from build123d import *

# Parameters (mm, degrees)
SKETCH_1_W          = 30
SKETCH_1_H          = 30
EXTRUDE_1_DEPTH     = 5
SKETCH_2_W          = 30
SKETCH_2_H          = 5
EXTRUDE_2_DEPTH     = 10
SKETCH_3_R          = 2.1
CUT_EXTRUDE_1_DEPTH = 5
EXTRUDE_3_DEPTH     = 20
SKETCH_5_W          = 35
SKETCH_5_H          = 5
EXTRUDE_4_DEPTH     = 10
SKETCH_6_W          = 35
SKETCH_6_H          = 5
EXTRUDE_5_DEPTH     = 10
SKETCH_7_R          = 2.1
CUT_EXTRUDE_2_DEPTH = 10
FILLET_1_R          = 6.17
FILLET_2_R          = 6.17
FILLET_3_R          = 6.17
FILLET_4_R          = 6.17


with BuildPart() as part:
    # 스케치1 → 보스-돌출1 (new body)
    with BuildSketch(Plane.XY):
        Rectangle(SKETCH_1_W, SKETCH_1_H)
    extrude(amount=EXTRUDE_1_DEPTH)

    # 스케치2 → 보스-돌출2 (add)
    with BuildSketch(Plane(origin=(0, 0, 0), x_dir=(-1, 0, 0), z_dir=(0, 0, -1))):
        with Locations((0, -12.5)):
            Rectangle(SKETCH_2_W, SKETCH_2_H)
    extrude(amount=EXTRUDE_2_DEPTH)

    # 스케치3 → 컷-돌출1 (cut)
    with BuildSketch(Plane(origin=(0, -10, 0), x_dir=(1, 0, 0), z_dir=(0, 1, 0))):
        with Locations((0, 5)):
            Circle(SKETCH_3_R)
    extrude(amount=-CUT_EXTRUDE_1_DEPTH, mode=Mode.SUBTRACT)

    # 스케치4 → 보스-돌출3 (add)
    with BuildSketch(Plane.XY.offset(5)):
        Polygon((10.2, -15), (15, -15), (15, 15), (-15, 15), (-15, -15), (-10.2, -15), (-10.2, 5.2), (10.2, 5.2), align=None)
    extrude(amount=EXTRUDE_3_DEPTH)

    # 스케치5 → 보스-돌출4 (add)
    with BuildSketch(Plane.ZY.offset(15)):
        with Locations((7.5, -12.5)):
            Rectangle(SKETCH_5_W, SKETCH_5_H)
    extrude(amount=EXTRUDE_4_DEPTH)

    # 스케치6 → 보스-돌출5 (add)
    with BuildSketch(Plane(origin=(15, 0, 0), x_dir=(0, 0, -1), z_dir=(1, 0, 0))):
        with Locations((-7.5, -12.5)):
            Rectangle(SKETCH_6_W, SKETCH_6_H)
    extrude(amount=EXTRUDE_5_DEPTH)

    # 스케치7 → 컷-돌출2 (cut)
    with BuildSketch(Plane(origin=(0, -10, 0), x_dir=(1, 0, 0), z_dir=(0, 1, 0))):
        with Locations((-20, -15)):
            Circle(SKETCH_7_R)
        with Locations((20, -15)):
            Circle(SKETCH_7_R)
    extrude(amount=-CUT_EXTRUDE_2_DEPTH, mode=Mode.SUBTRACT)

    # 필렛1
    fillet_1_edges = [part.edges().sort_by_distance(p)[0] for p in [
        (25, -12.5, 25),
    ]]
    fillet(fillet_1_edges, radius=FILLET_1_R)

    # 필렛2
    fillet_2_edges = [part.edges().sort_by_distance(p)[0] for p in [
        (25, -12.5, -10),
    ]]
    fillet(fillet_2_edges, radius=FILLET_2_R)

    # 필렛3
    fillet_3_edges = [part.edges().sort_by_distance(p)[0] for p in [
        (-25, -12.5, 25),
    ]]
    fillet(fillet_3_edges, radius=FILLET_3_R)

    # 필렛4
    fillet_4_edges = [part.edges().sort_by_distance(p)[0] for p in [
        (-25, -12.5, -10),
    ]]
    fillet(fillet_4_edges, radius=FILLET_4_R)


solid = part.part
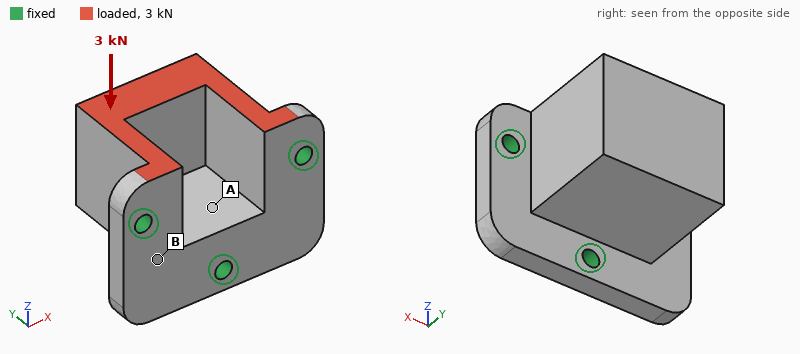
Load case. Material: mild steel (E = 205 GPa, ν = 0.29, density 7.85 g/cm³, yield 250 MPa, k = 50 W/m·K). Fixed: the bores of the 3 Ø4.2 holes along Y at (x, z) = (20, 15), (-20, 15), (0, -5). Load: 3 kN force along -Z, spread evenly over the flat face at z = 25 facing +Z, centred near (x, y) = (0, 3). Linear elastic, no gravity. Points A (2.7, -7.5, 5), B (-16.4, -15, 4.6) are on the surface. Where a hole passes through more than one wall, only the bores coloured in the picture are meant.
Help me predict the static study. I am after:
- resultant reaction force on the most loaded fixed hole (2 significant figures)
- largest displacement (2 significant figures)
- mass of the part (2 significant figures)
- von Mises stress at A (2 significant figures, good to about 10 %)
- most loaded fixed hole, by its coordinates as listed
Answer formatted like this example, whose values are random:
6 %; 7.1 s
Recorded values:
2.3 kN; 20 µm; 150 g; 28 MPa; (0, -5)
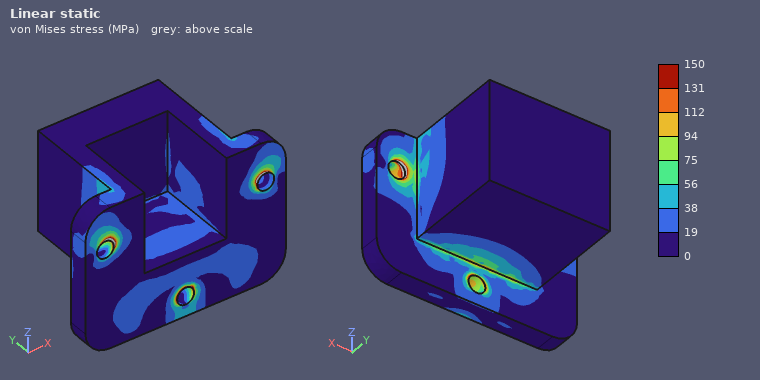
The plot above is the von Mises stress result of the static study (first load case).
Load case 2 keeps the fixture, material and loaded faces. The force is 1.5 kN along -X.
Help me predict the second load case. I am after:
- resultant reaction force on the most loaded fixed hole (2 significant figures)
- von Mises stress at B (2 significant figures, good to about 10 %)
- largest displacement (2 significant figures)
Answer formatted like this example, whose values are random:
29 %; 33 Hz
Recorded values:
910 N; 9.8 MPa; 15 µm
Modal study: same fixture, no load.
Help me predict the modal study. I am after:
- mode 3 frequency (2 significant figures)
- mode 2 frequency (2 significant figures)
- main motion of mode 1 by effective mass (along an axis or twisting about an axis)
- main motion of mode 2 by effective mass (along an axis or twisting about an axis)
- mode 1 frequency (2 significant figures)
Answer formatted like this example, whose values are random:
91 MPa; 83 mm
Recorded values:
13 kHz; 7400 Hz; along Z; along X; 6700 Hz
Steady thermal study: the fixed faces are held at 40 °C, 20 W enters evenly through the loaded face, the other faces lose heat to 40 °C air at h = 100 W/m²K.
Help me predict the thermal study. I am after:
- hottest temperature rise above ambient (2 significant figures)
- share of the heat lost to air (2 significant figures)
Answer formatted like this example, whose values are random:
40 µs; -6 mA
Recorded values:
25 K; 34 %
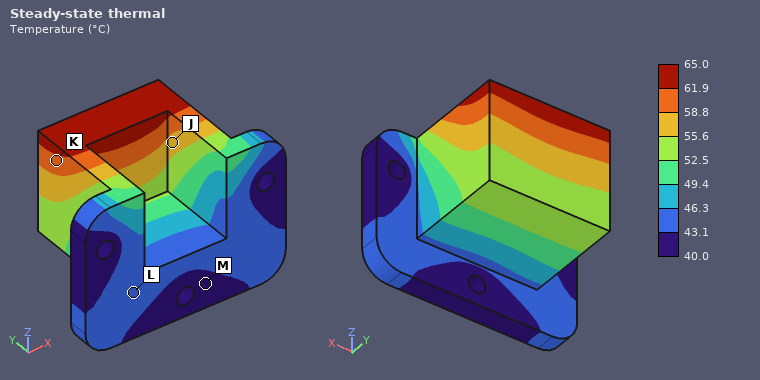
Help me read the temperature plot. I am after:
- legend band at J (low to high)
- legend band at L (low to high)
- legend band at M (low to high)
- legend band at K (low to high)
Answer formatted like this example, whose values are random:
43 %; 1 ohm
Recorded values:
55.6 to 58.8 °C; 43.1 to 46.3 °C; 40.0 to 43.1 °C; 58.8 to 61.9 °C
